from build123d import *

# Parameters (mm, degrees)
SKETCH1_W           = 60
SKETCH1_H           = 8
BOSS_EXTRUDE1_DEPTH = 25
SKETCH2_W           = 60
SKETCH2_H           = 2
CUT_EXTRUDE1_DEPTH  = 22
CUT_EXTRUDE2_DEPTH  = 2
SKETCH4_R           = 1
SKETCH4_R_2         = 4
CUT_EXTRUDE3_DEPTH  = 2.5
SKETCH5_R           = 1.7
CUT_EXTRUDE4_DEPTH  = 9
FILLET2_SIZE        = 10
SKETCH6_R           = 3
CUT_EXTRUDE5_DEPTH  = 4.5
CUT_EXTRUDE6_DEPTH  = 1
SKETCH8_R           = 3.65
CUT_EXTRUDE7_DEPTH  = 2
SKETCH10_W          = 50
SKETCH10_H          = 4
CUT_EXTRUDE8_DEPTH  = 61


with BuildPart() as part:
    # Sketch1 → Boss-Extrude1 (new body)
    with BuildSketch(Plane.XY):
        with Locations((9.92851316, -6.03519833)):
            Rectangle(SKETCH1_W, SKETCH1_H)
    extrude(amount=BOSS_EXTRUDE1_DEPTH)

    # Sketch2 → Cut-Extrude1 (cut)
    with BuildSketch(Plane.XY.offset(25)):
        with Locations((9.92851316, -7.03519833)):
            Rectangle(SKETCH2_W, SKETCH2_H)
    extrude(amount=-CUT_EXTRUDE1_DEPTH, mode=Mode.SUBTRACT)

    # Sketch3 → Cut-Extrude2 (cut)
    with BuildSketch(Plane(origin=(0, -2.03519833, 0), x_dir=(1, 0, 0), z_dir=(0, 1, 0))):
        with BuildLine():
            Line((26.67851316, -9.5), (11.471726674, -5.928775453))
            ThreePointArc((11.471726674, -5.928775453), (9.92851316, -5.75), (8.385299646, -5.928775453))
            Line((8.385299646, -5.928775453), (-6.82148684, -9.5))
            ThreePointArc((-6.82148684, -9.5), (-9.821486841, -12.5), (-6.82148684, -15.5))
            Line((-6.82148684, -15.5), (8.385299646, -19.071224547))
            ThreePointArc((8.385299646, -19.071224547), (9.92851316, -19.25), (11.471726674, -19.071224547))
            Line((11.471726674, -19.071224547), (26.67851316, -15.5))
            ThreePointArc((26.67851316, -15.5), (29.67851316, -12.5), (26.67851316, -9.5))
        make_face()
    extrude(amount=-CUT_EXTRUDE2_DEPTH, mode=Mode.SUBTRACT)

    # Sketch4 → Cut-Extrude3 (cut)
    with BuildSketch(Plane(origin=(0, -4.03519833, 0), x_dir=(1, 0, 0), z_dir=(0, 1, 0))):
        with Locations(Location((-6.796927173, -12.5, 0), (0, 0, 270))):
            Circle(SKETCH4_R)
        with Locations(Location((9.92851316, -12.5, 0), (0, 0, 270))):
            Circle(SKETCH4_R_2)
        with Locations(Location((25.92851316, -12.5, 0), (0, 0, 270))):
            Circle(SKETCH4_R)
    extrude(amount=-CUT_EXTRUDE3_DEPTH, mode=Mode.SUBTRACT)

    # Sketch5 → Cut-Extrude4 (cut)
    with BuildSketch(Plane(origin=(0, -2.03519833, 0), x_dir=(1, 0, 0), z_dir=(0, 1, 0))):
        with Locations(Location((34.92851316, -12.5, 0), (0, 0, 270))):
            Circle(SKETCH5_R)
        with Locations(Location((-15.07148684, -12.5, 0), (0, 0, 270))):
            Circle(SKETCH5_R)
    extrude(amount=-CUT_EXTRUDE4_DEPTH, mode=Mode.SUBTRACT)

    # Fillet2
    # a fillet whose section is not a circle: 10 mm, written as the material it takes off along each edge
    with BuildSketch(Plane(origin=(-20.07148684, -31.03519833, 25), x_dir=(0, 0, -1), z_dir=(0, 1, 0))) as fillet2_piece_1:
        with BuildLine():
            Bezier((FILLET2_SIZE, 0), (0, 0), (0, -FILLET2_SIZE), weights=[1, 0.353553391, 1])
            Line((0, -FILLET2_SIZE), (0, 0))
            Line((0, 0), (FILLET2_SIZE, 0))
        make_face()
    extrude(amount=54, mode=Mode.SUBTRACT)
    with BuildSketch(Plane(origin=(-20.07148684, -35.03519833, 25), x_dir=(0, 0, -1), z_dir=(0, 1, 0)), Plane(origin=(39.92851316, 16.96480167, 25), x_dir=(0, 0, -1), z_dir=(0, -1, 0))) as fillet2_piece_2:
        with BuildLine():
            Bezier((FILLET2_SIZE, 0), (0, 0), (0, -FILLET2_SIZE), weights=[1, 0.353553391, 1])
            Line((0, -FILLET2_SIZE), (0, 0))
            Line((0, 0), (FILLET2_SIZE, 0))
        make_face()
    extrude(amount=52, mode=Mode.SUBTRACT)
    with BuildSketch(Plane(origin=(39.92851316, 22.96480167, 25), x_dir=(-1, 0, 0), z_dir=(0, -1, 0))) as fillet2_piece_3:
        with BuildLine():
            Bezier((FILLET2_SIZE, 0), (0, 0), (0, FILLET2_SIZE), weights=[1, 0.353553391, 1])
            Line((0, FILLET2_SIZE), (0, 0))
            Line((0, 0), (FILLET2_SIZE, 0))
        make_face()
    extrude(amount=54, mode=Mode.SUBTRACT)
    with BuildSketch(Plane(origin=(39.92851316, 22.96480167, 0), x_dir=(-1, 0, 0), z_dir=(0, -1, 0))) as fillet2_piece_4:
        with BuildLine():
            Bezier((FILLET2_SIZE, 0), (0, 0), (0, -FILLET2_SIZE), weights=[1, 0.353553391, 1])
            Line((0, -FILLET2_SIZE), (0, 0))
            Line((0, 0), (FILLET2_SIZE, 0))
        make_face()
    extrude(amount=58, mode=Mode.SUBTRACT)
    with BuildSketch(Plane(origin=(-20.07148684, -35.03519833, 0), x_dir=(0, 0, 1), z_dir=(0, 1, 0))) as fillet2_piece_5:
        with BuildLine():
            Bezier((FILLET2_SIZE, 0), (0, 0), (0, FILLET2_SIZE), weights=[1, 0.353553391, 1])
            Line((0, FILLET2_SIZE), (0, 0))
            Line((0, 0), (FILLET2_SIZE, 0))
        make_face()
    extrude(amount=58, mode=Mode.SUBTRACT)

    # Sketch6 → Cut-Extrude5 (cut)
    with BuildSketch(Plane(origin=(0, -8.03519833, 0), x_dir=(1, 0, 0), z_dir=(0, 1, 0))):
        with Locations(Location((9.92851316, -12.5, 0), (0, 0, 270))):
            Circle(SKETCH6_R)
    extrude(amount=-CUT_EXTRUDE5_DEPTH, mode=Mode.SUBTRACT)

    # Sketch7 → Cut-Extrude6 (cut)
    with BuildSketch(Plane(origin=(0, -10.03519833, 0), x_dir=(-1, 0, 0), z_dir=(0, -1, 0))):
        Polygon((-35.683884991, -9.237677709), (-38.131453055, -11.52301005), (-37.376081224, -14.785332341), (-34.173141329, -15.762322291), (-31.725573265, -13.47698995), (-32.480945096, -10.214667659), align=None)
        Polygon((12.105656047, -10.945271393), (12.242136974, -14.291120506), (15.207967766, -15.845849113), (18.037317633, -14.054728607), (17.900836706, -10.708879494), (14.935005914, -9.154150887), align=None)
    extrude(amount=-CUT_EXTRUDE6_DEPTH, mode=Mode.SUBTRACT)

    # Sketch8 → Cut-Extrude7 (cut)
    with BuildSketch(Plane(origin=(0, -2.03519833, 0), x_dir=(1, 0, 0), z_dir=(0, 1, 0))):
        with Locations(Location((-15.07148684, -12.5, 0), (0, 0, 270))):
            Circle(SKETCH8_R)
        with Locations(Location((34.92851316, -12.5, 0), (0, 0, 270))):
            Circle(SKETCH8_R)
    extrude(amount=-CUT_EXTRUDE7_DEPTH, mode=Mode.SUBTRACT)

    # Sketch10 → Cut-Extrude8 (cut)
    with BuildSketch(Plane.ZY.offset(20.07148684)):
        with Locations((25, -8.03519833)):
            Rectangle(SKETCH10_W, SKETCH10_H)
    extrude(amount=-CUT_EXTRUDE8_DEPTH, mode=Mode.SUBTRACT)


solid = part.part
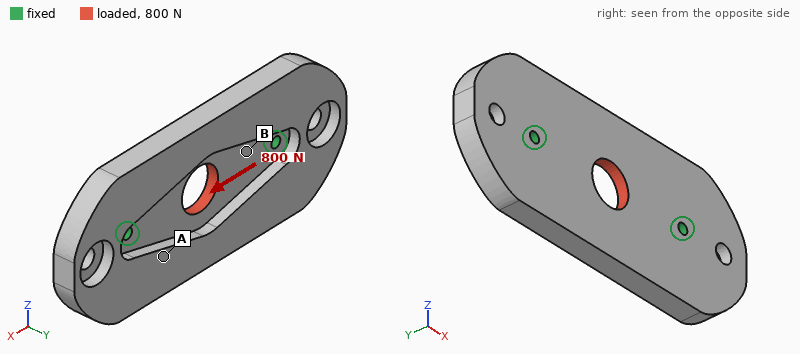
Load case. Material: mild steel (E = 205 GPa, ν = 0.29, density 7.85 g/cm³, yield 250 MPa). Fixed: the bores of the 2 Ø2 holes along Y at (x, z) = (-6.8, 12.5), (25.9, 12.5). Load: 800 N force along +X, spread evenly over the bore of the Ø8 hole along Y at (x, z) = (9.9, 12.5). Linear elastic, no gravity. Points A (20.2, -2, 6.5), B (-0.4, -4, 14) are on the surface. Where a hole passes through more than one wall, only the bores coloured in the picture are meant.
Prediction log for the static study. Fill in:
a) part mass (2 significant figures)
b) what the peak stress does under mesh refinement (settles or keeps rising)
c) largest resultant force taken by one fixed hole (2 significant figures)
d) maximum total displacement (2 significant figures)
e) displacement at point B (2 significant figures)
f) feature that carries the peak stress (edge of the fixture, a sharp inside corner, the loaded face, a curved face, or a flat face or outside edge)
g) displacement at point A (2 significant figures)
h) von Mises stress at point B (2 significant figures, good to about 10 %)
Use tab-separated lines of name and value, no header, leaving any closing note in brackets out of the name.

part mass	35 g
what the peak stress does under mesh refinement	keeps rising
largest resultant force taken by one fixed hole	400 N
maximum total displacement	1.3 µm
displacement at point B	0.66 µm
feature that carries the peak stress	edge of the fixture
displacement at point A	0.73 µm
von Mises stress at point B	15 MPa
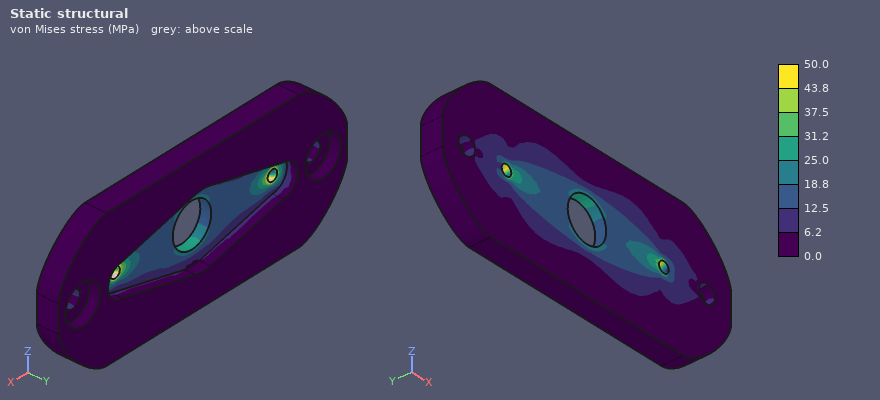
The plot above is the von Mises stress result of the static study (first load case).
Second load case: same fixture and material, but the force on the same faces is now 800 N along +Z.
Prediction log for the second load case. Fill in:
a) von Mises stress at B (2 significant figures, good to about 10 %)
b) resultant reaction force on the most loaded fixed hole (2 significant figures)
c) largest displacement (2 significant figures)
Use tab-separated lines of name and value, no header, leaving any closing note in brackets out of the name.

von Mises stress at B	18 MPa
resultant reaction force on the most loaded fixed hole	410 N
largest displacement	2.5 µm
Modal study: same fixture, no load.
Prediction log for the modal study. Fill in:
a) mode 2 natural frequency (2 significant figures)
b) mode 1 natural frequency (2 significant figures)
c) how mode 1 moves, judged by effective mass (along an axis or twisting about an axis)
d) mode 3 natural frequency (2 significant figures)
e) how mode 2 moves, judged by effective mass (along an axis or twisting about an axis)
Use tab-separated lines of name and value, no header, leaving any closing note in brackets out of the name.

mode 2 natural frequency	7800 Hz
mode 1 natural frequency	5100 Hz
how mode 1 moves, judged by effective mass	twisting about X
mode 3 natural frequency	9500 Hz
how mode 2 moves, judged by effective mass	along Y
